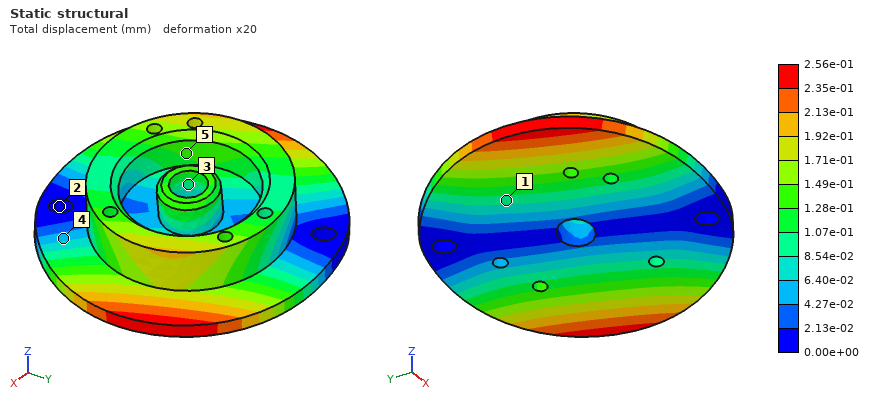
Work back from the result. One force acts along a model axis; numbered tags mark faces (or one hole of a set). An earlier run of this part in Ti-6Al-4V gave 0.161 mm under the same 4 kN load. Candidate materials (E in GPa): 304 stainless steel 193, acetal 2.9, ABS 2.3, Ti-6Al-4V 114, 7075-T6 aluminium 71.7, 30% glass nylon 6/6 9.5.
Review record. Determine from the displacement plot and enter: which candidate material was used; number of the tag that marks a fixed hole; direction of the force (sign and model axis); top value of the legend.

7075-T6 aluminium
2
+X
2.56e-01 mm
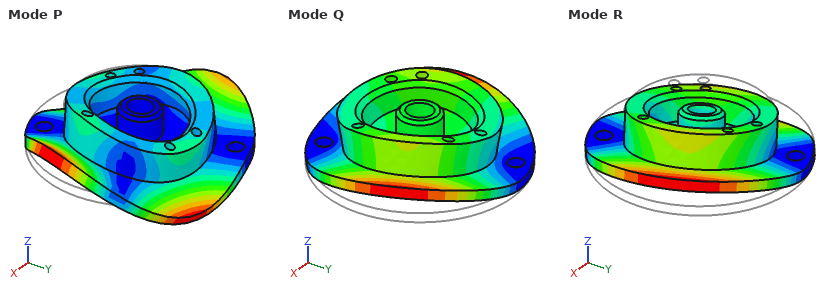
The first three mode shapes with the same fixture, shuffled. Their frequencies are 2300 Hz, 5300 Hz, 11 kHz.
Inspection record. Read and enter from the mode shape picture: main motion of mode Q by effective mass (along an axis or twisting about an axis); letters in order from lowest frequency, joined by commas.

along Z
R, Q, P
